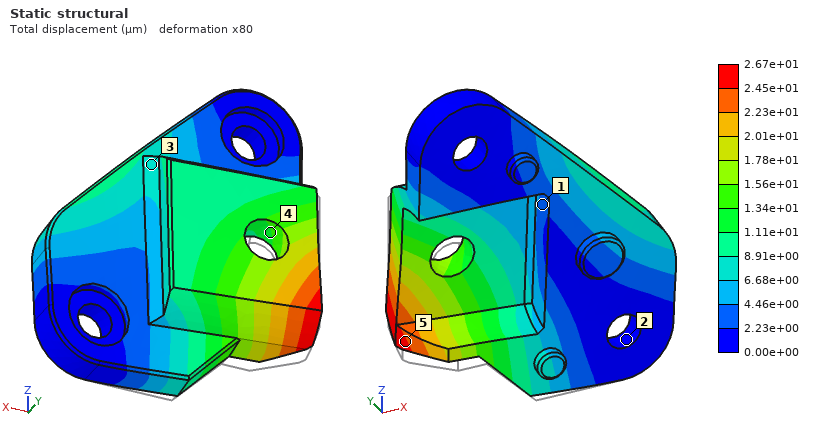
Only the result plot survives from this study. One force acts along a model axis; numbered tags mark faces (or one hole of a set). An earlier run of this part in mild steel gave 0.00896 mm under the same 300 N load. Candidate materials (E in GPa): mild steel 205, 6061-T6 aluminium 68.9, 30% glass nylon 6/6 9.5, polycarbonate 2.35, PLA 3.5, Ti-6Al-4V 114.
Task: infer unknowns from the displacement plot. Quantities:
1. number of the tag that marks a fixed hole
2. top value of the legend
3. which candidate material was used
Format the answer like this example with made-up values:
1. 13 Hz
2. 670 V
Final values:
1. 2
2. 2.67e+01 µm
3. 6061-T6 aluminium
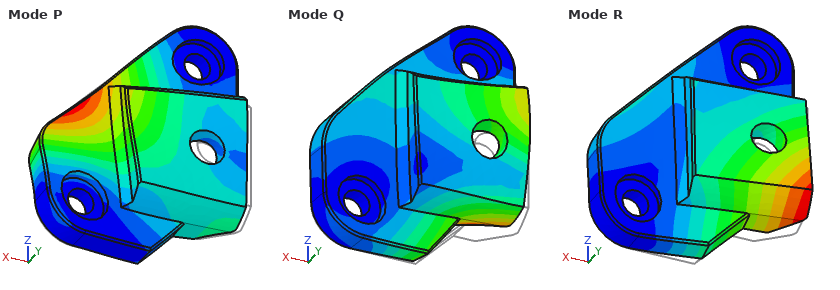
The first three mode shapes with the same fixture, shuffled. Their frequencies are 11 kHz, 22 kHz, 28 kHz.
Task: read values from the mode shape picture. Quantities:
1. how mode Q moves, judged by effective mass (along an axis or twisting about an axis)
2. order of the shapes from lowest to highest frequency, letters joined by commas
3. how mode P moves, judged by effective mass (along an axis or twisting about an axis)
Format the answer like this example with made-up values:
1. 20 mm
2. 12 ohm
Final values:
1. along Z
2. R, P, Q
3. along Y
